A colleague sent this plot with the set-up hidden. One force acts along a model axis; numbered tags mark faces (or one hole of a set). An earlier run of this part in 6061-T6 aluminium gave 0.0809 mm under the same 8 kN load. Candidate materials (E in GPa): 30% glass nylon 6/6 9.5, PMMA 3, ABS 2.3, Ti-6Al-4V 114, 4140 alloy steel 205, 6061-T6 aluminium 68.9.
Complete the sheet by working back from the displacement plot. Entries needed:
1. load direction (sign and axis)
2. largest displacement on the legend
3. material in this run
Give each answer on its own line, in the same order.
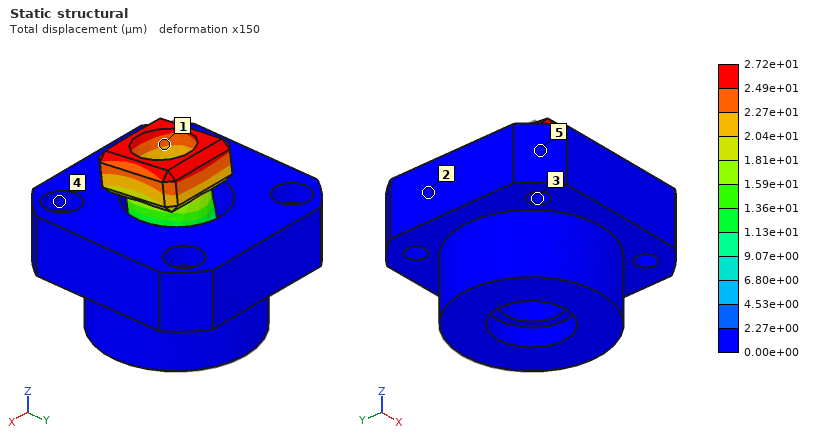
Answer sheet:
-Y
2.72e+01 µm
4140 alloy steel
